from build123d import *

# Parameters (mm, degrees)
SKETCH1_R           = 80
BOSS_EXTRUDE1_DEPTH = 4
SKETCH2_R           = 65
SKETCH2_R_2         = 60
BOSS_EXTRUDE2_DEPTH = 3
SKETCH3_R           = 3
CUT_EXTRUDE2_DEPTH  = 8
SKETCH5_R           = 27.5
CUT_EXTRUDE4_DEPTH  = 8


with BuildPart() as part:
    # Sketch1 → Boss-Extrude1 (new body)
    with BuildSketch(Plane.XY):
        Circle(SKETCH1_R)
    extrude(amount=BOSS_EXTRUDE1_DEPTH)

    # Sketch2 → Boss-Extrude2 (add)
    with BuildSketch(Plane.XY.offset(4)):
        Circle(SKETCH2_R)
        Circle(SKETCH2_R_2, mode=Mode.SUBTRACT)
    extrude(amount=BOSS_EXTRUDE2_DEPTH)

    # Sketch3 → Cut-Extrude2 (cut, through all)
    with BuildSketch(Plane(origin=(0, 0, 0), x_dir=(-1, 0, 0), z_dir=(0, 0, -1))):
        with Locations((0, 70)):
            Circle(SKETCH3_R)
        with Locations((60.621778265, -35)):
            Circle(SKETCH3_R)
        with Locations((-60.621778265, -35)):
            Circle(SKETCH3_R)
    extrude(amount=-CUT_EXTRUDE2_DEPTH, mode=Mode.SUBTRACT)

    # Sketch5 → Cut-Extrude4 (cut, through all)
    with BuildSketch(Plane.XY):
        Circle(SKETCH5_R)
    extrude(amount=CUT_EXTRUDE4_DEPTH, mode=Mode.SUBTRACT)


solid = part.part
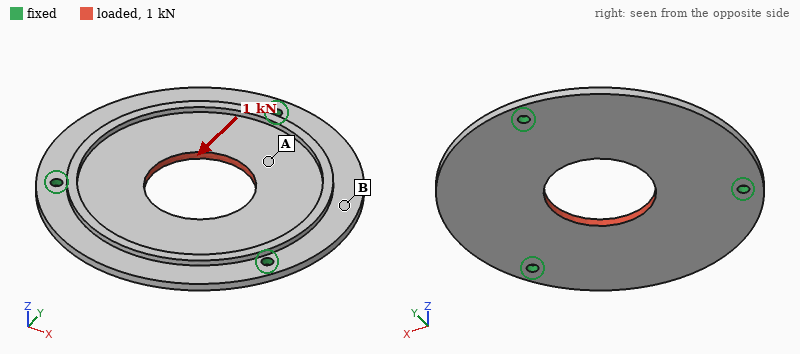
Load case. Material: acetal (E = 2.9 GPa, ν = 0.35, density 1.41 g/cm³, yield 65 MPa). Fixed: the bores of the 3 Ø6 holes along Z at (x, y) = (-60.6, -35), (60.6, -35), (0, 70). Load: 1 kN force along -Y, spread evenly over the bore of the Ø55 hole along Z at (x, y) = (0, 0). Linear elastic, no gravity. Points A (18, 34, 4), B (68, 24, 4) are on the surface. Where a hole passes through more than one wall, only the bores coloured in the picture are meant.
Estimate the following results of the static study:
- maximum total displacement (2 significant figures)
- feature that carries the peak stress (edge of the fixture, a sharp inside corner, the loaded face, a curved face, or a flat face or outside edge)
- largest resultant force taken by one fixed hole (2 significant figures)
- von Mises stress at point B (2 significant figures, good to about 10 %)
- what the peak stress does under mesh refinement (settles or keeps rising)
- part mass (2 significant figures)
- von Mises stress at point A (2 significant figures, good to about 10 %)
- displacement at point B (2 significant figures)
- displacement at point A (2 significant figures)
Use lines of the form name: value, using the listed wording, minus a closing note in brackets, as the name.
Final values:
maximum total displacement: 78 µm
feature that carries the peak stress: edge of the fixture
largest resultant force taken by one fixed hole: 350 N
von Mises stress at point B: 0.85 MPa
what the peak stress does under mesh refinement: keeps rising
part mass: 110 g
von Mises stress at point A: 2.0 MPa
displacement at point B: 31 µm
displacement at point A: 36 µm
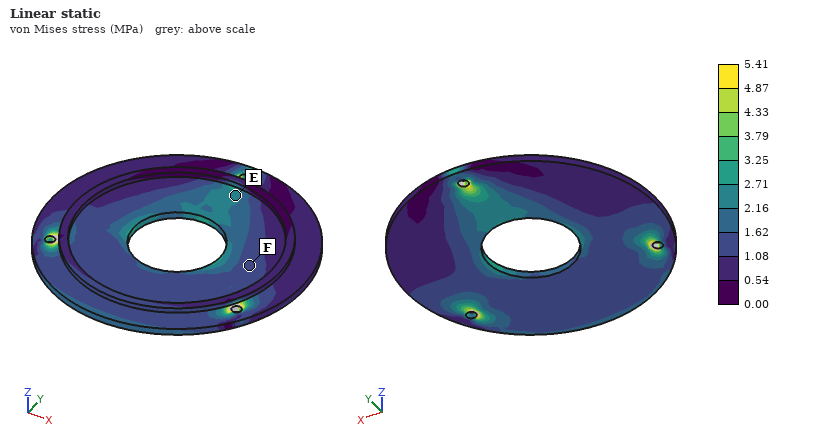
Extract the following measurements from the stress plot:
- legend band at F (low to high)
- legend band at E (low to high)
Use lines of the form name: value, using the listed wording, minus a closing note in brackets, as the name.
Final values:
legend band at F: 1.08 to 1.62 MPa
legend band at E: 2.16 to 2.71 MPa
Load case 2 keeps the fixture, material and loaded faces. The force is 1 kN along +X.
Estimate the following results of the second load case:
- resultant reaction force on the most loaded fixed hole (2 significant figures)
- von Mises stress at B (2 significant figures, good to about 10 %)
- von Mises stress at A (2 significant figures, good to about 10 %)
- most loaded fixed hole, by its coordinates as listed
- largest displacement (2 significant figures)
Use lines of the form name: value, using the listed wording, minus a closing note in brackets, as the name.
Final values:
resultant reaction force on the most loaded fixed hole: 360 N
von Mises stress at B: 1.3 MPa
von Mises stress at A: 1.2 MPa
most loaded fixed hole, by its coordinates as listed: (0, 70)
largest displacement: 71 µm
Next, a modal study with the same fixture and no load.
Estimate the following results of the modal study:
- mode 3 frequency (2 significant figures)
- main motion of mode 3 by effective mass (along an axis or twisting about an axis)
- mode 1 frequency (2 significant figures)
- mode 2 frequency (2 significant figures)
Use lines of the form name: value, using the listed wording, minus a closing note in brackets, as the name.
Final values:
mode 3 frequency: 380 Hz
main motion of mode 3 by effective mass: along Z
mode 1 frequency: 310 Hz
mode 2 frequency: 310 Hz
